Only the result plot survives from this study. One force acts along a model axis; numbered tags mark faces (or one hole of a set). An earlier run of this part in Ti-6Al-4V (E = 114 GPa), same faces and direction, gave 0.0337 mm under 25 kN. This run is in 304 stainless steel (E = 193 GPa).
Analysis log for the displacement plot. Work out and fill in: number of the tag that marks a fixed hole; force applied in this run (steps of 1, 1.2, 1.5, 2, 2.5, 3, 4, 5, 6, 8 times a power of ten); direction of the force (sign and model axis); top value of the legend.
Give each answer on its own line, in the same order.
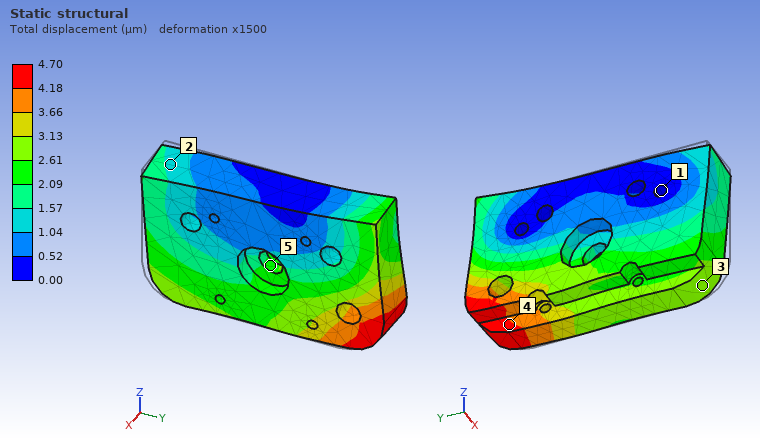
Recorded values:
1
6 kN
+Y
4.70 µm
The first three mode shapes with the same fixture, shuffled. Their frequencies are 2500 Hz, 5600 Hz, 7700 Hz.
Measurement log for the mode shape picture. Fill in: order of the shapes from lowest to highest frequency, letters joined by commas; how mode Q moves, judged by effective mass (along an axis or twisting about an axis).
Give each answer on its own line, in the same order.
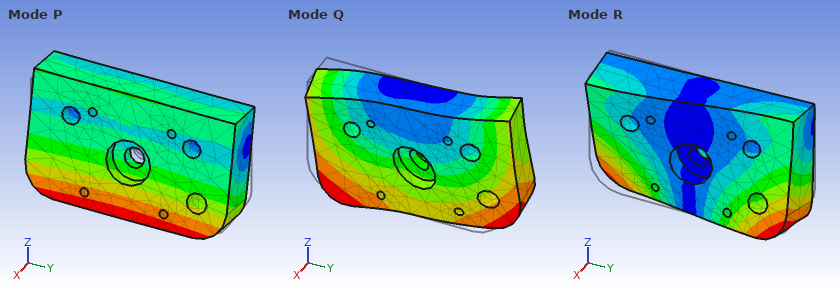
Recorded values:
P, R, Q
along Y
